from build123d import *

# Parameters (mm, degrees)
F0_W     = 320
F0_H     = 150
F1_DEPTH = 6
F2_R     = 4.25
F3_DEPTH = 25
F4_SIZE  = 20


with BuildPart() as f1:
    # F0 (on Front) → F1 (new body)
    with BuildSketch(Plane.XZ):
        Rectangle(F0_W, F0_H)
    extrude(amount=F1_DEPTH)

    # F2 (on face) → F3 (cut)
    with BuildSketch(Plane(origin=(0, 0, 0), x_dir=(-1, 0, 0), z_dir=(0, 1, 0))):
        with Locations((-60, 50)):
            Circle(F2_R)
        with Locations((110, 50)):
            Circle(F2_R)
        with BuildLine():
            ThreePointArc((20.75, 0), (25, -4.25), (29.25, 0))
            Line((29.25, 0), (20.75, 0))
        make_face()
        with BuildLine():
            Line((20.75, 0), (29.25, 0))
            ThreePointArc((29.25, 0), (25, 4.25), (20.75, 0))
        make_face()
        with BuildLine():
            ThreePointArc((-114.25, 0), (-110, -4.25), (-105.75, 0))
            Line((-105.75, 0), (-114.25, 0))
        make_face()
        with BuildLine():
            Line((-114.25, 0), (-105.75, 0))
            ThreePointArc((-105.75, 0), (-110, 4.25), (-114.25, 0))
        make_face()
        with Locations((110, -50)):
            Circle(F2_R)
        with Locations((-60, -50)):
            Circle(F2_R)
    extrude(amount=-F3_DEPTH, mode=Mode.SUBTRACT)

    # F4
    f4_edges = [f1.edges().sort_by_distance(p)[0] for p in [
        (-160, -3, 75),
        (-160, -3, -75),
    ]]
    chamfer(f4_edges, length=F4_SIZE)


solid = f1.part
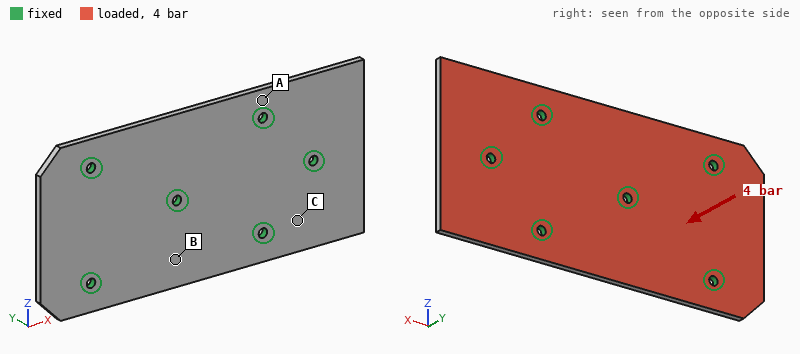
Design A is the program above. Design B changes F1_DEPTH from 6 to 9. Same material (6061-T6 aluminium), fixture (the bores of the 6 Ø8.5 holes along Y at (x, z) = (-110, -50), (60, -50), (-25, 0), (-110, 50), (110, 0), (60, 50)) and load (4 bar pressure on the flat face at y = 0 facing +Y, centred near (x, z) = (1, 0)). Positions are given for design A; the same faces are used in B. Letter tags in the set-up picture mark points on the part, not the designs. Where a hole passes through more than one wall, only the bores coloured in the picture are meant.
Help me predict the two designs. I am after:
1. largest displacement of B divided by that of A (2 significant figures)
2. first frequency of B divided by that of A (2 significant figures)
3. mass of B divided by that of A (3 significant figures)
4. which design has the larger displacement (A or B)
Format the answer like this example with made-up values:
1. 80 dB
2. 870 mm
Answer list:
1. 0.31
2. 1.4
3. 1.50
4. A
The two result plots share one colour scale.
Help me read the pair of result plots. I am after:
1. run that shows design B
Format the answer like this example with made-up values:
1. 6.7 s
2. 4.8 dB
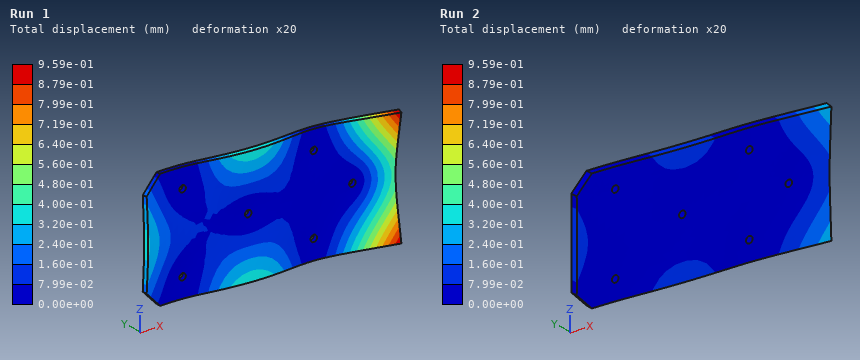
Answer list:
1. Run 2
